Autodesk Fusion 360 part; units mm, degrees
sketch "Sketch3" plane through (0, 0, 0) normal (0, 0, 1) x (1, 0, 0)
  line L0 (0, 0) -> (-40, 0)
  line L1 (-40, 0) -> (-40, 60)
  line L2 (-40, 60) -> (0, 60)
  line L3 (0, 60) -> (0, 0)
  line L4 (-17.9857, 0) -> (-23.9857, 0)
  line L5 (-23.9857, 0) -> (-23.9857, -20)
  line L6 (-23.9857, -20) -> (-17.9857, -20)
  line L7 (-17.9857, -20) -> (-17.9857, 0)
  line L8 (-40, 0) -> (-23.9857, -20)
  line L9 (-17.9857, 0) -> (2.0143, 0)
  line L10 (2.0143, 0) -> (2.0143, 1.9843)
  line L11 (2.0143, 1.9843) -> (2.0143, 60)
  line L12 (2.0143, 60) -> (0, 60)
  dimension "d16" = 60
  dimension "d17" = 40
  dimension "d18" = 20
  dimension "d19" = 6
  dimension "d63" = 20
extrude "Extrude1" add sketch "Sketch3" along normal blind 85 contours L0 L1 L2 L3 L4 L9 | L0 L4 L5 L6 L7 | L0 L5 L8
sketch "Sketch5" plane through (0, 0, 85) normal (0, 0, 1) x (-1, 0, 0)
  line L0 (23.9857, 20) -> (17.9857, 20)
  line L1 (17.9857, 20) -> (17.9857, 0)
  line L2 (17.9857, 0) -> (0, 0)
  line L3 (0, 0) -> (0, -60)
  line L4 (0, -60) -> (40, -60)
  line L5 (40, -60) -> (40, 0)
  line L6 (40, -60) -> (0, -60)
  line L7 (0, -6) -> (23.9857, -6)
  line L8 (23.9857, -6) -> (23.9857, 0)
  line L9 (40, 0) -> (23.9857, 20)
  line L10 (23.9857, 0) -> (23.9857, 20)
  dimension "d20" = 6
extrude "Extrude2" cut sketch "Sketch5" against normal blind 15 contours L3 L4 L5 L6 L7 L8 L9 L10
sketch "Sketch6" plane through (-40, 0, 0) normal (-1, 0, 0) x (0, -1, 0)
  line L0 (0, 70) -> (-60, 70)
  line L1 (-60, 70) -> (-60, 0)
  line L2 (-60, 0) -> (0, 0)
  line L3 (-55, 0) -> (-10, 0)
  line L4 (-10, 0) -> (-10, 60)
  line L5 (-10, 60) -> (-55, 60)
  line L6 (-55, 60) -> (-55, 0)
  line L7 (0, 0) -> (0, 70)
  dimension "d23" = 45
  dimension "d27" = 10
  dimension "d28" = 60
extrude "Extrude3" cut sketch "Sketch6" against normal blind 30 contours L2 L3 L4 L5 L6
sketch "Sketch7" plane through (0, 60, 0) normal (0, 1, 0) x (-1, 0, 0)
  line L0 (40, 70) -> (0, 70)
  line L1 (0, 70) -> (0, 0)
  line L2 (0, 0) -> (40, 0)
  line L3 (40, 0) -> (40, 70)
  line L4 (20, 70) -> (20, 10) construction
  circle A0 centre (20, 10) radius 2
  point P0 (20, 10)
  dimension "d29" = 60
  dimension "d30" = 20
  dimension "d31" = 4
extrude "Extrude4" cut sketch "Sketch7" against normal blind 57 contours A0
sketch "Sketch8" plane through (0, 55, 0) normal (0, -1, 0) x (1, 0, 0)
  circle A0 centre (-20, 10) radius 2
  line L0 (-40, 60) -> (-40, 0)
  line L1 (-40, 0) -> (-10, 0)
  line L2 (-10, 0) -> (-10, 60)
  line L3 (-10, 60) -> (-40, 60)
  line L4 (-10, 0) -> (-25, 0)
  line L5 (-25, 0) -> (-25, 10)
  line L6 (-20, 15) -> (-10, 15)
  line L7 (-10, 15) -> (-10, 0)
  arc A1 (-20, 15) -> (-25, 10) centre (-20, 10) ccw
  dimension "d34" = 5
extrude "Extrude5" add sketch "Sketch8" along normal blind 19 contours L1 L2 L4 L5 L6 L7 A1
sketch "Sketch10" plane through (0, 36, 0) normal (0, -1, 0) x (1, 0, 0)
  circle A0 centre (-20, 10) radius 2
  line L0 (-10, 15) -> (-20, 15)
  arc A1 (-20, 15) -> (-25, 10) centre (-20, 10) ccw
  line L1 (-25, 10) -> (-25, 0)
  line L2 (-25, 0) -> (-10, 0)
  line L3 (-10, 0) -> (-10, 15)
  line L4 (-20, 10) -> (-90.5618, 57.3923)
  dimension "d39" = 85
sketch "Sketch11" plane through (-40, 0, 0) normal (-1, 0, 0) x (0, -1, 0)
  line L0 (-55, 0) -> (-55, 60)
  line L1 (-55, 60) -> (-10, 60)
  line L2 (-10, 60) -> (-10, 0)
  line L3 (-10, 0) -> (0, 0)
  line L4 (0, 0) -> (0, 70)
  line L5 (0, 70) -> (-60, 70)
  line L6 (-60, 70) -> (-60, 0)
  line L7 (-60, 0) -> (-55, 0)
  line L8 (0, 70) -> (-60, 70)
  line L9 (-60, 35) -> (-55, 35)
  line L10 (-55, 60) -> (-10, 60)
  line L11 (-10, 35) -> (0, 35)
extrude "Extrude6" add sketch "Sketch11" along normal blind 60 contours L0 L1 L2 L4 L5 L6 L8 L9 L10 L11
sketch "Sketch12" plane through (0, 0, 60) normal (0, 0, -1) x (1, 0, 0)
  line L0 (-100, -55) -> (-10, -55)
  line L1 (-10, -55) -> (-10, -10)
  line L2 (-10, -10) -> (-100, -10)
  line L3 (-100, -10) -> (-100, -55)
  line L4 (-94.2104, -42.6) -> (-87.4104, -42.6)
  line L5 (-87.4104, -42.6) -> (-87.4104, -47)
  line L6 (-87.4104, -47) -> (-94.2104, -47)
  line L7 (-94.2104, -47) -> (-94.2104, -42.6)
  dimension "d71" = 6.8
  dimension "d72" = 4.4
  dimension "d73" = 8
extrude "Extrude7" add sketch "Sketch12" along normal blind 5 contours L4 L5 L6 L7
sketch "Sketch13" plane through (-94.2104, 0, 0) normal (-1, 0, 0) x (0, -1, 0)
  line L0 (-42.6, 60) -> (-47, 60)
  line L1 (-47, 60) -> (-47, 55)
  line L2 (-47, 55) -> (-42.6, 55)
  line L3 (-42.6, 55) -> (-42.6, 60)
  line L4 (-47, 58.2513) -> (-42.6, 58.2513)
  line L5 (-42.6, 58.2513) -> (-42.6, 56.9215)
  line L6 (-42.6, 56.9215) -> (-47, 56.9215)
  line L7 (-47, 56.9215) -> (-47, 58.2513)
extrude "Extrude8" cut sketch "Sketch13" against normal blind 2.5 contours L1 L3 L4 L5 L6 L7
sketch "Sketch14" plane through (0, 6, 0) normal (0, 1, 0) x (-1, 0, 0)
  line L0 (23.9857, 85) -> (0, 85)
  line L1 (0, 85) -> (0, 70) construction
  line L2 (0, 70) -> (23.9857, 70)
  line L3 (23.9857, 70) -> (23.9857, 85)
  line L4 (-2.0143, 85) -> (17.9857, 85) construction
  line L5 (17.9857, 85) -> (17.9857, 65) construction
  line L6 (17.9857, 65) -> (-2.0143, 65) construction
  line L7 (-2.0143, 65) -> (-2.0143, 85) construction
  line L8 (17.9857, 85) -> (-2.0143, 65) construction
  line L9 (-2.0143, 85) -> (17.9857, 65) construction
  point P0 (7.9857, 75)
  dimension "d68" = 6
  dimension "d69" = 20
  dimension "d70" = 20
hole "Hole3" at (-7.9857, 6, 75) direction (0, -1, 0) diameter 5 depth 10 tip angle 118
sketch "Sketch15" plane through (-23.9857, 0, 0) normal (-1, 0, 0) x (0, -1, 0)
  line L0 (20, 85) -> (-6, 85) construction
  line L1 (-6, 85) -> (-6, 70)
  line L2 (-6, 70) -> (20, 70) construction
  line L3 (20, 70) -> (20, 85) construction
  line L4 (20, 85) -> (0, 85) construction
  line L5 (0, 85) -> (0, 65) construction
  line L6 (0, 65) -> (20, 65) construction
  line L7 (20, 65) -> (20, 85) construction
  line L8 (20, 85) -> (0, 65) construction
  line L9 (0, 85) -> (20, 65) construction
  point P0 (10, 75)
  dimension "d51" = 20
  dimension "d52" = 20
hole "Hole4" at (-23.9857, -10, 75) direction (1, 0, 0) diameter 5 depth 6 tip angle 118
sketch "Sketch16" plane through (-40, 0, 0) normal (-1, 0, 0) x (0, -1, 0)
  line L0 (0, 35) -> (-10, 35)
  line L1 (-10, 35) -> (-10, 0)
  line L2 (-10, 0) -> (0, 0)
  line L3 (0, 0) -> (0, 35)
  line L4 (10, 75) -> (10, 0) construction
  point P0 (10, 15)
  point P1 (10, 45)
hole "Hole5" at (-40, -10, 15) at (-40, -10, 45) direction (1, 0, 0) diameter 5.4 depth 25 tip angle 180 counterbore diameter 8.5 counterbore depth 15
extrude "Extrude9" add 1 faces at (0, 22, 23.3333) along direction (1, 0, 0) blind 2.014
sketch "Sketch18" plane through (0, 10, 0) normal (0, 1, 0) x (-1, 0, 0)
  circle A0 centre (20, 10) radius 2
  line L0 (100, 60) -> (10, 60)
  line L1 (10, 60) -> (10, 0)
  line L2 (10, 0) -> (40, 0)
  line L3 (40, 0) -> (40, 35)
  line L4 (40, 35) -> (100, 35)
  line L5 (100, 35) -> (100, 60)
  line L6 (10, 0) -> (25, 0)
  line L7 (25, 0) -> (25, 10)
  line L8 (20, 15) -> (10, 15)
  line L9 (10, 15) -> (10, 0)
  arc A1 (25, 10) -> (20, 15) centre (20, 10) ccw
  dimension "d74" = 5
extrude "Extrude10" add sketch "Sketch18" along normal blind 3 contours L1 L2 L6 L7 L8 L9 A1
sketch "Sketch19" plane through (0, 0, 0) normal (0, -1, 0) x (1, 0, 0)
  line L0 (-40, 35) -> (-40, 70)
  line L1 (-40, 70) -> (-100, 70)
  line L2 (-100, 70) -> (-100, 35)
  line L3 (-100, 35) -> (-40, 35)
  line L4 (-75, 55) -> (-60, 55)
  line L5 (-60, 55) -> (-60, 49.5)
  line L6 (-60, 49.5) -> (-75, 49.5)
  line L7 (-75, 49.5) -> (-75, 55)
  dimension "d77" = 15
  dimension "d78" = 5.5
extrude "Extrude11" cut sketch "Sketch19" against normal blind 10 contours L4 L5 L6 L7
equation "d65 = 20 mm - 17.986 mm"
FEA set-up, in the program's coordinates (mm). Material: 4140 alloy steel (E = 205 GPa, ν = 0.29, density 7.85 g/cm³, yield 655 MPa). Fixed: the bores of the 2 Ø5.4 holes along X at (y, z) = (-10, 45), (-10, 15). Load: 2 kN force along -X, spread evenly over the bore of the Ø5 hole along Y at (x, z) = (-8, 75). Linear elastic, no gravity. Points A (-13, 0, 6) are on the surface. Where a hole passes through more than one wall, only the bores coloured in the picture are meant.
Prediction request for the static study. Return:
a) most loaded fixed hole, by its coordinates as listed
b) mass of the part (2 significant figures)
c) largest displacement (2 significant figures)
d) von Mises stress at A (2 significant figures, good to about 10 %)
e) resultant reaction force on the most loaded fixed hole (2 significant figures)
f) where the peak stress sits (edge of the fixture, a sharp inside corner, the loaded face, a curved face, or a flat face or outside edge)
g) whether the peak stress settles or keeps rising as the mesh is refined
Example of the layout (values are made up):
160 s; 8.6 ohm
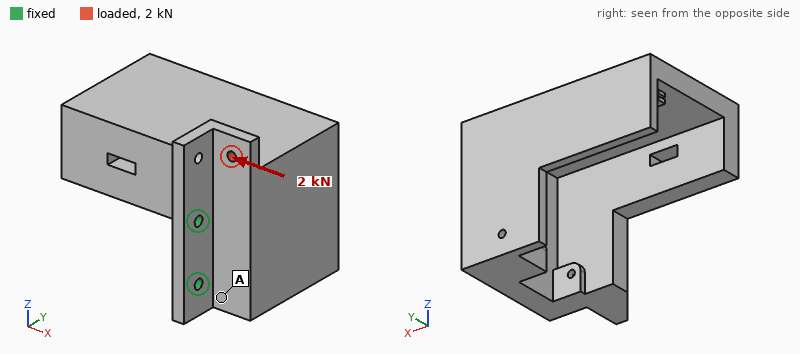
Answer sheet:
(-10, 45); 1.4 kg; 49 µm; 11 MPa; 3.6 kN; edge of the fixture; keeps rising
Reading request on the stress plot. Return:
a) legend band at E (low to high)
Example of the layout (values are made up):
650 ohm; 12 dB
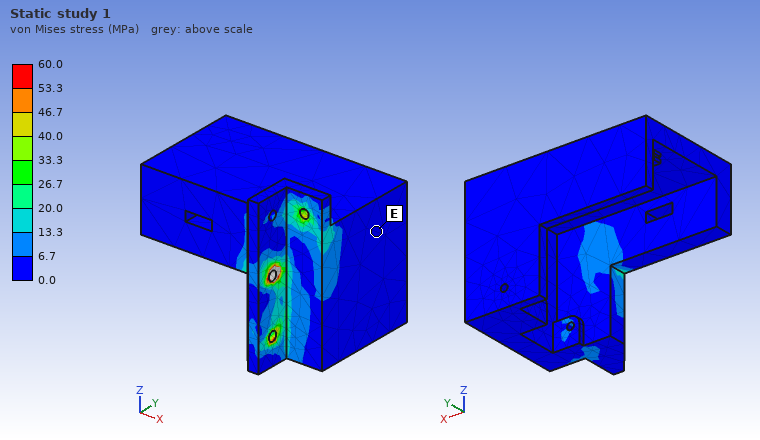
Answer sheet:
0.0 to 6.7 MPa
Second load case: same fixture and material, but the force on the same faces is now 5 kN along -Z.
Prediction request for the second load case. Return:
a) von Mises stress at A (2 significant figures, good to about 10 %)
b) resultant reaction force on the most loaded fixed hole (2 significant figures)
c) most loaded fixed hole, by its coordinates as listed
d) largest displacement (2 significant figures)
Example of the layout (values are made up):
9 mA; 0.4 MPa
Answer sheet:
16 MPa; 4.1 kN; (-10, 45); 22 µm
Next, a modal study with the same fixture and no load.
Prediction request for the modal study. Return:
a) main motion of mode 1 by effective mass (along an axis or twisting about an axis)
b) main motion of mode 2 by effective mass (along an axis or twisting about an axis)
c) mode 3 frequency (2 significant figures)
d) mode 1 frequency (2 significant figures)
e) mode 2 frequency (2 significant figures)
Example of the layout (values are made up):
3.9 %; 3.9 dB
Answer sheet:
along X; along Z; 2500 Hz; 670 Hz; 1500 Hz
